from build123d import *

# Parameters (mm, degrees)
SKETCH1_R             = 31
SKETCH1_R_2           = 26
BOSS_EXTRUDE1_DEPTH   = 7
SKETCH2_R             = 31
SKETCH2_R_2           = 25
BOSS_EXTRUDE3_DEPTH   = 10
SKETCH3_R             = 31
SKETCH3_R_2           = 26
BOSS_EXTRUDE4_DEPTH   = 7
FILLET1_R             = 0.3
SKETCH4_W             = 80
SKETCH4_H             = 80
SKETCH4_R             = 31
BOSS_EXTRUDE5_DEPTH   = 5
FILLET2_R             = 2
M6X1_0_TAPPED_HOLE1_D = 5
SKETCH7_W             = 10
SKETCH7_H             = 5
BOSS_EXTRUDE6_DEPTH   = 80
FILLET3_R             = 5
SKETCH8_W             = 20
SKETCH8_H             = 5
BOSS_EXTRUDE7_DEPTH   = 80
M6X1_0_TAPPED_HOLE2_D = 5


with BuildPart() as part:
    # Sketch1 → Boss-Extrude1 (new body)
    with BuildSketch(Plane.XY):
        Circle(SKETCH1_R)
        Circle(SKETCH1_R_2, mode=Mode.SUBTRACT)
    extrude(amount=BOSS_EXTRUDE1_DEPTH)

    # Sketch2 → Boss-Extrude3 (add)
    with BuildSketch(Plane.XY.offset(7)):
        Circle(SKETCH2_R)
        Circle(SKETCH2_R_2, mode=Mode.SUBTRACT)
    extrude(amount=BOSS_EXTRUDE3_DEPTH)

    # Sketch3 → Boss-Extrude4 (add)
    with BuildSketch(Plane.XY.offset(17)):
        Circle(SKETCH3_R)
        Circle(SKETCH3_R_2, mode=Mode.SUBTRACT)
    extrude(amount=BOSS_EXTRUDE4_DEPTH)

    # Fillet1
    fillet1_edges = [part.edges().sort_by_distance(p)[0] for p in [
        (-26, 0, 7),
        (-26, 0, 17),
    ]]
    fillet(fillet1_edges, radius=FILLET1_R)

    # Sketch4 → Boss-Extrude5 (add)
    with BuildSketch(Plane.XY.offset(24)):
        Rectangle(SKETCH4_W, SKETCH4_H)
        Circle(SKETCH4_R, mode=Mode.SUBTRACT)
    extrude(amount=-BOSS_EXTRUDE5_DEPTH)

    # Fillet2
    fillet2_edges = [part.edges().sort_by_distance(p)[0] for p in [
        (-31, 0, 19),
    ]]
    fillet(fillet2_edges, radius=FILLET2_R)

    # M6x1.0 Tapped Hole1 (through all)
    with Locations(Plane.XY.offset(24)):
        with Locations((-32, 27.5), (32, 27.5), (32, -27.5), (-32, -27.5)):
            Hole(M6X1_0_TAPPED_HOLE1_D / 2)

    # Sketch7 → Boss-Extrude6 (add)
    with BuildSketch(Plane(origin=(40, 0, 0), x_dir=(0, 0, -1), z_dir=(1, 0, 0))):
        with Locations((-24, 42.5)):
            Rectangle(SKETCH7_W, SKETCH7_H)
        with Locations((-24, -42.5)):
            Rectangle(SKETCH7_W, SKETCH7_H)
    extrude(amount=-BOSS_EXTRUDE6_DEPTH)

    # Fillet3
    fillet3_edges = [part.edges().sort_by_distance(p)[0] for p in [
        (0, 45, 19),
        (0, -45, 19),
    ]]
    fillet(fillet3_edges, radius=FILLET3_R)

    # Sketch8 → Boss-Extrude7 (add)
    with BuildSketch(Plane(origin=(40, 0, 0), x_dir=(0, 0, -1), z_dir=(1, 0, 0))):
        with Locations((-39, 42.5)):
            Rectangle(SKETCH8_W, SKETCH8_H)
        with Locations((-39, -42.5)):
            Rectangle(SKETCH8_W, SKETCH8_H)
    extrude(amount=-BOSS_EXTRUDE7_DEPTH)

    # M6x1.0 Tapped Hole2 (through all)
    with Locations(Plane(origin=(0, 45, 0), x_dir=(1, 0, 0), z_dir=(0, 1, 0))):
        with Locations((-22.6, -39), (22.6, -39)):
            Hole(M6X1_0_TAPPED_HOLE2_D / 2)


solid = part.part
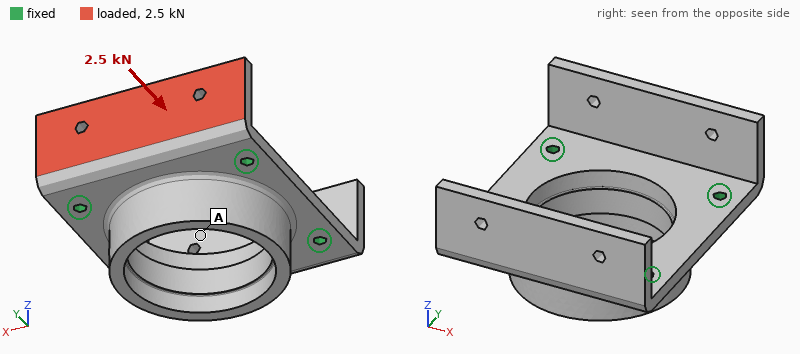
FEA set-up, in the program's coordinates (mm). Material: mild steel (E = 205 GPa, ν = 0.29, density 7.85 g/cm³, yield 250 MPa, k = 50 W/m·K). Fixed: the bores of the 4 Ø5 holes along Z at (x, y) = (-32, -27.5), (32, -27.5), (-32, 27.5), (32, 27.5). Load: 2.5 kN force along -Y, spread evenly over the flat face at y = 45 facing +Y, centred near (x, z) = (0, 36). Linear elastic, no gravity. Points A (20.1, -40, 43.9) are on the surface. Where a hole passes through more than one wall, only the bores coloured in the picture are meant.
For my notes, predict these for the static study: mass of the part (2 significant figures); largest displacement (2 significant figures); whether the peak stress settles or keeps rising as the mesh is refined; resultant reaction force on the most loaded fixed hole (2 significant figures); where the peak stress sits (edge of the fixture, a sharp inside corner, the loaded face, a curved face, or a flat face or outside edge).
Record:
490 g
0.13 mm
keeps rising
1.3 kN
edge of the fixture
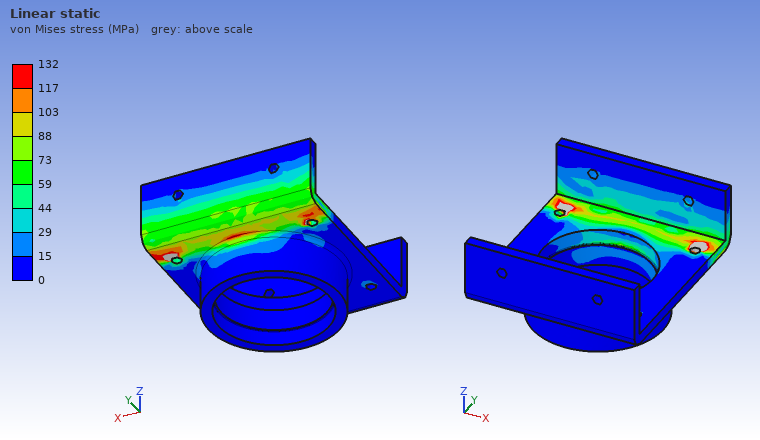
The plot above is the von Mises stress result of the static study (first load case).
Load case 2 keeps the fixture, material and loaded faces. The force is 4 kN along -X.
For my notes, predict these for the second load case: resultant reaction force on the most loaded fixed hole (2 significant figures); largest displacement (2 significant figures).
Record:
2.4 kN
24 µm
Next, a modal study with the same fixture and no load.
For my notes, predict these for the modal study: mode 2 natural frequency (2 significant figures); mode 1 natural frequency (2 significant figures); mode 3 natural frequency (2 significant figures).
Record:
2900 Hz
2900 Hz
4600 Hz
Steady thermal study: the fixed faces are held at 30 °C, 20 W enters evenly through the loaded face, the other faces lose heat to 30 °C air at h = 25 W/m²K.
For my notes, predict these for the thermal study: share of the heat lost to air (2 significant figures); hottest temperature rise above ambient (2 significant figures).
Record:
20 %
32 K
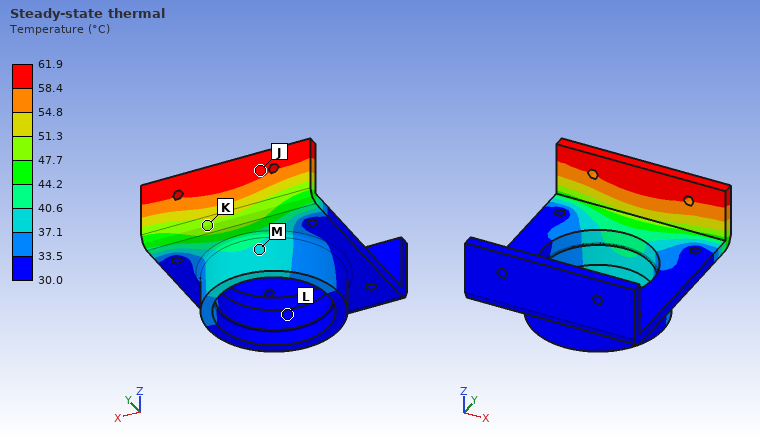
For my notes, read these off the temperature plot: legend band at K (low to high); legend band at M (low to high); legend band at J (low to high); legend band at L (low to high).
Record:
47.7 to 51.3 °C
37.1 to 40.6 °C
58.4 to 61.9 °C
30.0 to 33.5 °C
